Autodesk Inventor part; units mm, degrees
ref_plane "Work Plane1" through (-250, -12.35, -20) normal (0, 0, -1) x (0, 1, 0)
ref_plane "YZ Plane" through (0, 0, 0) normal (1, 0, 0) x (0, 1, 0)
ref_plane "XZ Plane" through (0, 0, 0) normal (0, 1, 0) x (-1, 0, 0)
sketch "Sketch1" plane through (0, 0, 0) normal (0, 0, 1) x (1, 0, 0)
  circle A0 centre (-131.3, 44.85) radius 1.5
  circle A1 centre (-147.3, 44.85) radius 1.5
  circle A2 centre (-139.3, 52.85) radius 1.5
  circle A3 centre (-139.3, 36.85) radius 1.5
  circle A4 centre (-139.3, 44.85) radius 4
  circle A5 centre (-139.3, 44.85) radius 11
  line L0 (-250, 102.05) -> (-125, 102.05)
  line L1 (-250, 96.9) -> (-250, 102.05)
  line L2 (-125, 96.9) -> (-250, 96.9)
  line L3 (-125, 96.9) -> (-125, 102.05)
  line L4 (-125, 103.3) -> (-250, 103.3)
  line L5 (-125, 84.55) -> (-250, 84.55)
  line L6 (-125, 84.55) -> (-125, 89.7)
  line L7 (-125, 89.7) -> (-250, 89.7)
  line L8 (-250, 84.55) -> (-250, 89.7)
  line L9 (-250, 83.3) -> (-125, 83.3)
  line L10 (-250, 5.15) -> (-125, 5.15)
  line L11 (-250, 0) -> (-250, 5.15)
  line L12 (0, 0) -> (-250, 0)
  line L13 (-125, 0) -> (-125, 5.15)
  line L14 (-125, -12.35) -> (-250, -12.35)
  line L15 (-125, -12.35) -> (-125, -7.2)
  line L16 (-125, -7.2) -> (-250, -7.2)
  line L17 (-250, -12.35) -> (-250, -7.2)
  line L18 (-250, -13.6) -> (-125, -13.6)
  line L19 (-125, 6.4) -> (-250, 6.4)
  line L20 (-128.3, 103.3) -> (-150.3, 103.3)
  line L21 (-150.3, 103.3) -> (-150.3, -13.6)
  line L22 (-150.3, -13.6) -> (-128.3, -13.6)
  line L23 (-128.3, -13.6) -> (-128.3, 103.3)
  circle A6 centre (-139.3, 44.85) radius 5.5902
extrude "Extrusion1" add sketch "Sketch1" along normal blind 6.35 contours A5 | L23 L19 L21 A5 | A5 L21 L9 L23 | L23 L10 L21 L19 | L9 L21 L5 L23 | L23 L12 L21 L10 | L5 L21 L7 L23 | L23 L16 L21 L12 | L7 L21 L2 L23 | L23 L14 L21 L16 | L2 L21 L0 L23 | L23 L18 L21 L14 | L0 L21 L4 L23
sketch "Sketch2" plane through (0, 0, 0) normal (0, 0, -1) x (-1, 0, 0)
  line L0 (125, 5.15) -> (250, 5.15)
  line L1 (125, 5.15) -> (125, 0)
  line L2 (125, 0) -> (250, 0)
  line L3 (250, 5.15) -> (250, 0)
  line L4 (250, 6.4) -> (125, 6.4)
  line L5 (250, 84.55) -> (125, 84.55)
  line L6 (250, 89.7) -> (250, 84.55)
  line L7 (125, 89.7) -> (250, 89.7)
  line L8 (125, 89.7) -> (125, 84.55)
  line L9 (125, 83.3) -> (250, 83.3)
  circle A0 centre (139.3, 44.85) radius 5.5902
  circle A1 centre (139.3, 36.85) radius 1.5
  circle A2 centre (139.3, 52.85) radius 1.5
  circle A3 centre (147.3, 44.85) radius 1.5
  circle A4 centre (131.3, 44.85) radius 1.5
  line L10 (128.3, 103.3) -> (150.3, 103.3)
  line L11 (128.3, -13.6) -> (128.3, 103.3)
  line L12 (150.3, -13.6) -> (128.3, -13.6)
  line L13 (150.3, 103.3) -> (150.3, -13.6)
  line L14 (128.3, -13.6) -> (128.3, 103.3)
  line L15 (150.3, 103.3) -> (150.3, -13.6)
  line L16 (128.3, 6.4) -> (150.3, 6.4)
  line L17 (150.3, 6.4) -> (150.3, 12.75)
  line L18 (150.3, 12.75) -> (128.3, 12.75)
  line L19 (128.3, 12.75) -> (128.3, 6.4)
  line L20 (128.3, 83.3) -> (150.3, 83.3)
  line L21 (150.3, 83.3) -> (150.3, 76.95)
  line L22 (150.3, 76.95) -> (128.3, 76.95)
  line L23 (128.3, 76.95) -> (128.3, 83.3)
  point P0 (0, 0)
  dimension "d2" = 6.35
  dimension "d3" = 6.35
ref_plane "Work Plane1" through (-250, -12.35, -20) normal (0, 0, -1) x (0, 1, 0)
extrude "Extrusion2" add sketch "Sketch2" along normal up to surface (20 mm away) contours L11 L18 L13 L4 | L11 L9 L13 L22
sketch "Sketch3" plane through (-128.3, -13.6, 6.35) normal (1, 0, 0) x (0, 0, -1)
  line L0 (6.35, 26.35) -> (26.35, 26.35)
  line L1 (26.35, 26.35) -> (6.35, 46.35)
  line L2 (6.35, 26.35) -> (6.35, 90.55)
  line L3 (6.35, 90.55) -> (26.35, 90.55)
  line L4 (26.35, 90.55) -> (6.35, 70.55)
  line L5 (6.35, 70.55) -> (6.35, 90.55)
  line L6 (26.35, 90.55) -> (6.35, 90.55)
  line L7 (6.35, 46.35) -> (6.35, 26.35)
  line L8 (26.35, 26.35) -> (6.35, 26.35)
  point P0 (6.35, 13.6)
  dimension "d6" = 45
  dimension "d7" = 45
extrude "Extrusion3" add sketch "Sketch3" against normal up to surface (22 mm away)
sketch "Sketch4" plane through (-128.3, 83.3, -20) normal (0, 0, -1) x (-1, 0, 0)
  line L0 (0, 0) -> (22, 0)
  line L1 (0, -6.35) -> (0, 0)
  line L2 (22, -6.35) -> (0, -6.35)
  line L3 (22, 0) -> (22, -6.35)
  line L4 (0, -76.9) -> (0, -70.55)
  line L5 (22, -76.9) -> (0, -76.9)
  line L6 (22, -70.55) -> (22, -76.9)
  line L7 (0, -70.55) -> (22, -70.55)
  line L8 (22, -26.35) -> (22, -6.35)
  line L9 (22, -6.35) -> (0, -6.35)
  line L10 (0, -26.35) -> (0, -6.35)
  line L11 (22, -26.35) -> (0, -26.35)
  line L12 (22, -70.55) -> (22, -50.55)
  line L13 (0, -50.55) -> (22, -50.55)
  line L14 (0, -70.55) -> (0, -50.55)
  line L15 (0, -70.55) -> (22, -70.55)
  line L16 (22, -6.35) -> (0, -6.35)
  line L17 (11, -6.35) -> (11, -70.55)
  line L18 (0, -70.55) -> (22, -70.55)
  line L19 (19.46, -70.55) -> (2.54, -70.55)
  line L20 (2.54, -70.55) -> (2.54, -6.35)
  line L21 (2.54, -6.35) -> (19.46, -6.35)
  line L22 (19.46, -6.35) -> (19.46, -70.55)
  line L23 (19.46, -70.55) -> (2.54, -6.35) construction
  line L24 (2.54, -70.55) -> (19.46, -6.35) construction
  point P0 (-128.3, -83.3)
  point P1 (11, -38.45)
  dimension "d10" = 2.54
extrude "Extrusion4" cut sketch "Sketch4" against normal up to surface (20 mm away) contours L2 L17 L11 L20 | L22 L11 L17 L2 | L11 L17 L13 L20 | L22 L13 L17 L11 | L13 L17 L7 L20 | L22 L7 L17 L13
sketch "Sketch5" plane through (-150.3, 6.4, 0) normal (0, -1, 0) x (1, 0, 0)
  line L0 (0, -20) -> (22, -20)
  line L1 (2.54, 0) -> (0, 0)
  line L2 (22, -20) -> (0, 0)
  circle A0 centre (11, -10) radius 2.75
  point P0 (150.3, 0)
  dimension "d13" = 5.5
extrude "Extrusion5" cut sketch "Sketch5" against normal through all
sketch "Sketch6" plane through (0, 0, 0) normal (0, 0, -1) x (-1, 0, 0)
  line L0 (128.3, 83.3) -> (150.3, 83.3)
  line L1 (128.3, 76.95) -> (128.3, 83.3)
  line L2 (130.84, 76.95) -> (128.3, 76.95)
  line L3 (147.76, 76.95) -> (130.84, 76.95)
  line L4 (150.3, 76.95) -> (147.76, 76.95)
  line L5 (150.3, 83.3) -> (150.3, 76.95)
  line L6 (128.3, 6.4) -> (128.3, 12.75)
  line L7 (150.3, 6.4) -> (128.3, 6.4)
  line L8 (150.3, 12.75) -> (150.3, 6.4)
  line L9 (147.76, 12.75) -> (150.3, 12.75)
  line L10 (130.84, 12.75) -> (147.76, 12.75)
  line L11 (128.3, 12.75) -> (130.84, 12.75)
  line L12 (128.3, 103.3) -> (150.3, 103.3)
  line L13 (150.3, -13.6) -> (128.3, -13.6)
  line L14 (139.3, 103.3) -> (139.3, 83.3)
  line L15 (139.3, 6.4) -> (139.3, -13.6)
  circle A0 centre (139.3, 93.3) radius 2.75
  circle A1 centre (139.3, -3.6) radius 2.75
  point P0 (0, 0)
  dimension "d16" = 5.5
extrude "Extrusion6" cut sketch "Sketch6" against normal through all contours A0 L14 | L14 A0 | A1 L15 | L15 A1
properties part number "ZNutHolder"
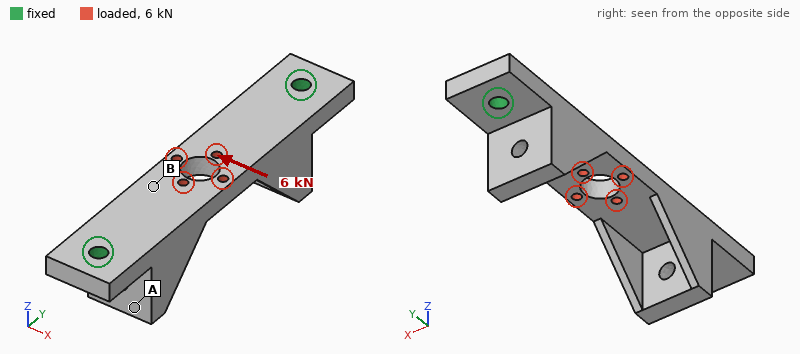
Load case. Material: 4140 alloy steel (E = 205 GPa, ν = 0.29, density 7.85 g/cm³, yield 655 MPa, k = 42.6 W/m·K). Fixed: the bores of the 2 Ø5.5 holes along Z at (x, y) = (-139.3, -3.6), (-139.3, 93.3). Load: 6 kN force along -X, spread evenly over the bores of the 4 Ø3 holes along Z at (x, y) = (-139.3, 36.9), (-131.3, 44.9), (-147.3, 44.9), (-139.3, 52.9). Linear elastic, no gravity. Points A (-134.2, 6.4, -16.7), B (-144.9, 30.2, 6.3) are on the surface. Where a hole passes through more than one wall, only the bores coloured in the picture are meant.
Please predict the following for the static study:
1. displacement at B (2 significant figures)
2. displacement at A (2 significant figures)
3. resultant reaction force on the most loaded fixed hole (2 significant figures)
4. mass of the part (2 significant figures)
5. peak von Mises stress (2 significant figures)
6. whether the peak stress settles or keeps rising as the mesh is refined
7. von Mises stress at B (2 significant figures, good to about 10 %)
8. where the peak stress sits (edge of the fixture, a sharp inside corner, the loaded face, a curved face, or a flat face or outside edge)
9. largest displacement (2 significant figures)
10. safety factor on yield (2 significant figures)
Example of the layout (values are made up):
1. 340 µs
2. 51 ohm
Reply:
1. 51 µm
2. 14 µm
3. 3.0 kN
4. 180 g
5. 540 MPa
6. settles
7. 70 MPa
8. the loaded face
9. 66 µm
10. 1.2
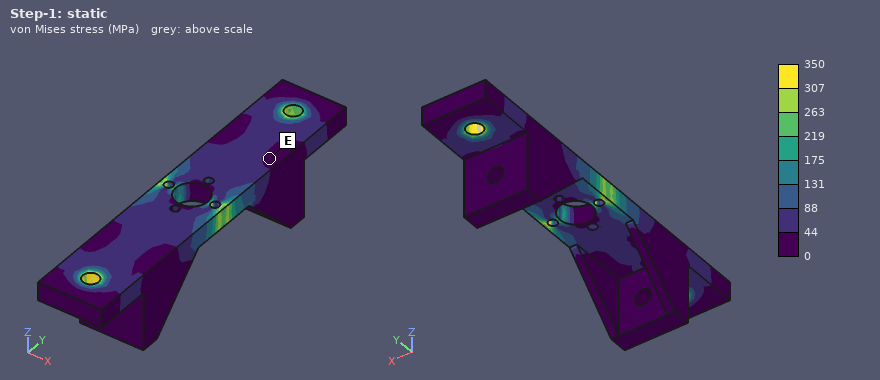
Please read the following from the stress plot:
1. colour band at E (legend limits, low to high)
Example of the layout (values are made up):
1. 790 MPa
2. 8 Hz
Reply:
1. 0 to 44 MPa
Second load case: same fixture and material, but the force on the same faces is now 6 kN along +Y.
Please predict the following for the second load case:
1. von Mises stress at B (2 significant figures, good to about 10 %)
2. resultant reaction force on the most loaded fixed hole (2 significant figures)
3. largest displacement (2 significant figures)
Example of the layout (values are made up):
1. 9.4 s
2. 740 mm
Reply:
1. 22 MPa
2. 3.0 kN
3. 5.8 µm
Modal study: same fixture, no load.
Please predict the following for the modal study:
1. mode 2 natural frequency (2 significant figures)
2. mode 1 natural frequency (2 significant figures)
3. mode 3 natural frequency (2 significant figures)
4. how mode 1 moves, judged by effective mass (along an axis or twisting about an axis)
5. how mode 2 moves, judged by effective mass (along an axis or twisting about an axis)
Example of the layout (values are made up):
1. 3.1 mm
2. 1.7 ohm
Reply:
1. 5600 Hz
2. 3000 Hz
3. 7000 Hz
4. along Z
5. along X
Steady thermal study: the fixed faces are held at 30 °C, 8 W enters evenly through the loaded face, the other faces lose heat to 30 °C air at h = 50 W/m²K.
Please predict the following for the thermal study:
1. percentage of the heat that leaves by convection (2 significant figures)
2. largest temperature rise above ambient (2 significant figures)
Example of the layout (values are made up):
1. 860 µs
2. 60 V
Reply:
1. 46 %
2. 20 K
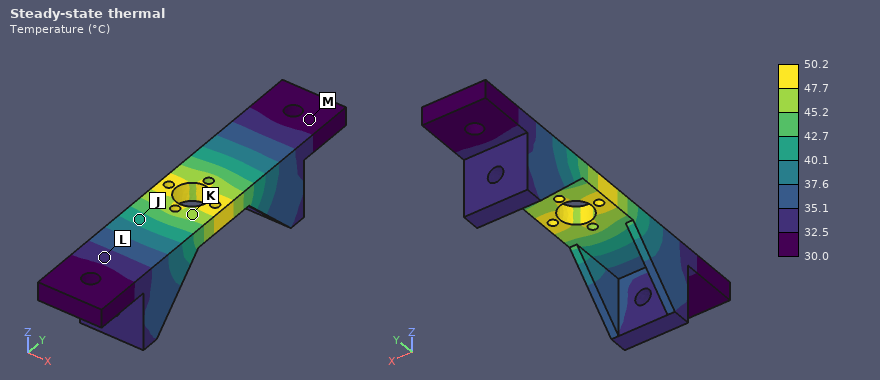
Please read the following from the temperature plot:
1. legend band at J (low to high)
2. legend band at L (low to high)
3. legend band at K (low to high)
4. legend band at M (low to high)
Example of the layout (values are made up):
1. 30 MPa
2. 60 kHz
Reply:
1. 40.1 to 42.7 °C
2. 32.5 to 35.1 °C
3. 45.2 to 47.7 °C
4. 30.0 to 32.5 °C
